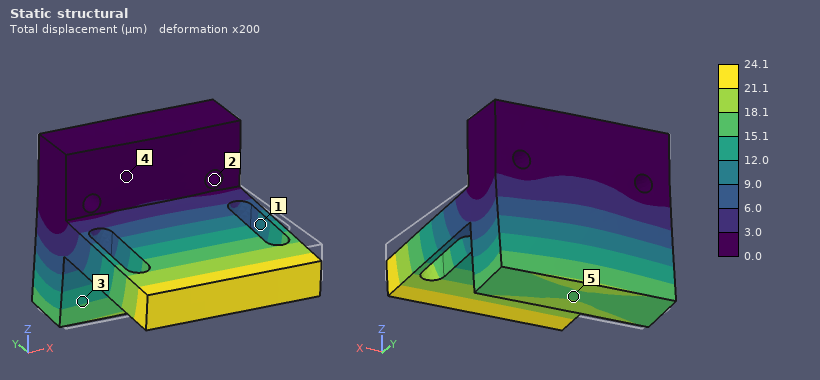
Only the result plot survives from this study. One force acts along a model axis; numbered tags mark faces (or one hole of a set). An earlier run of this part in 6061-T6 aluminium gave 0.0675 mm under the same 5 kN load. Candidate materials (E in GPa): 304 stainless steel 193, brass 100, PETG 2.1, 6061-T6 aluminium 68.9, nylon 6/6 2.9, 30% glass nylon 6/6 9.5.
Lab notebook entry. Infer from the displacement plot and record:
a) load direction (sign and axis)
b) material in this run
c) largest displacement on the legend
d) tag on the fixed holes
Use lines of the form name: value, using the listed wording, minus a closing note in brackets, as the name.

load direction: +Y
material in this run: 304 stainless steel
largest displacement on the legend: 24.1 µm
tag on the fixed holes: 2
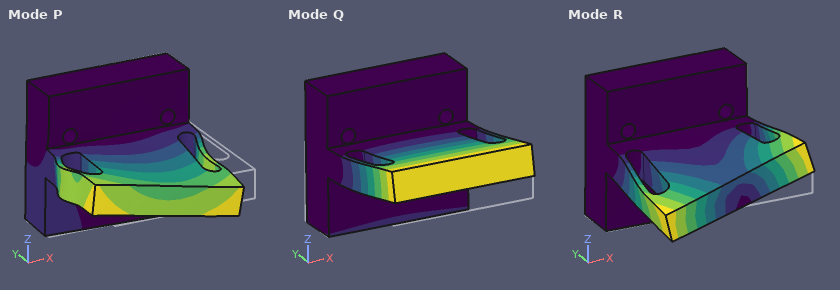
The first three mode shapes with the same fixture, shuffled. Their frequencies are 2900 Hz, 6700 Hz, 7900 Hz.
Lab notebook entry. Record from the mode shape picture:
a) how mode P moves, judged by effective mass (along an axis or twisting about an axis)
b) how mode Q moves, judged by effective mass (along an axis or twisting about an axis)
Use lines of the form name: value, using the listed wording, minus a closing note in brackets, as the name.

how mode P moves, judged by effective mass: along X
how mode Q moves, judged by effective mass: along Z
